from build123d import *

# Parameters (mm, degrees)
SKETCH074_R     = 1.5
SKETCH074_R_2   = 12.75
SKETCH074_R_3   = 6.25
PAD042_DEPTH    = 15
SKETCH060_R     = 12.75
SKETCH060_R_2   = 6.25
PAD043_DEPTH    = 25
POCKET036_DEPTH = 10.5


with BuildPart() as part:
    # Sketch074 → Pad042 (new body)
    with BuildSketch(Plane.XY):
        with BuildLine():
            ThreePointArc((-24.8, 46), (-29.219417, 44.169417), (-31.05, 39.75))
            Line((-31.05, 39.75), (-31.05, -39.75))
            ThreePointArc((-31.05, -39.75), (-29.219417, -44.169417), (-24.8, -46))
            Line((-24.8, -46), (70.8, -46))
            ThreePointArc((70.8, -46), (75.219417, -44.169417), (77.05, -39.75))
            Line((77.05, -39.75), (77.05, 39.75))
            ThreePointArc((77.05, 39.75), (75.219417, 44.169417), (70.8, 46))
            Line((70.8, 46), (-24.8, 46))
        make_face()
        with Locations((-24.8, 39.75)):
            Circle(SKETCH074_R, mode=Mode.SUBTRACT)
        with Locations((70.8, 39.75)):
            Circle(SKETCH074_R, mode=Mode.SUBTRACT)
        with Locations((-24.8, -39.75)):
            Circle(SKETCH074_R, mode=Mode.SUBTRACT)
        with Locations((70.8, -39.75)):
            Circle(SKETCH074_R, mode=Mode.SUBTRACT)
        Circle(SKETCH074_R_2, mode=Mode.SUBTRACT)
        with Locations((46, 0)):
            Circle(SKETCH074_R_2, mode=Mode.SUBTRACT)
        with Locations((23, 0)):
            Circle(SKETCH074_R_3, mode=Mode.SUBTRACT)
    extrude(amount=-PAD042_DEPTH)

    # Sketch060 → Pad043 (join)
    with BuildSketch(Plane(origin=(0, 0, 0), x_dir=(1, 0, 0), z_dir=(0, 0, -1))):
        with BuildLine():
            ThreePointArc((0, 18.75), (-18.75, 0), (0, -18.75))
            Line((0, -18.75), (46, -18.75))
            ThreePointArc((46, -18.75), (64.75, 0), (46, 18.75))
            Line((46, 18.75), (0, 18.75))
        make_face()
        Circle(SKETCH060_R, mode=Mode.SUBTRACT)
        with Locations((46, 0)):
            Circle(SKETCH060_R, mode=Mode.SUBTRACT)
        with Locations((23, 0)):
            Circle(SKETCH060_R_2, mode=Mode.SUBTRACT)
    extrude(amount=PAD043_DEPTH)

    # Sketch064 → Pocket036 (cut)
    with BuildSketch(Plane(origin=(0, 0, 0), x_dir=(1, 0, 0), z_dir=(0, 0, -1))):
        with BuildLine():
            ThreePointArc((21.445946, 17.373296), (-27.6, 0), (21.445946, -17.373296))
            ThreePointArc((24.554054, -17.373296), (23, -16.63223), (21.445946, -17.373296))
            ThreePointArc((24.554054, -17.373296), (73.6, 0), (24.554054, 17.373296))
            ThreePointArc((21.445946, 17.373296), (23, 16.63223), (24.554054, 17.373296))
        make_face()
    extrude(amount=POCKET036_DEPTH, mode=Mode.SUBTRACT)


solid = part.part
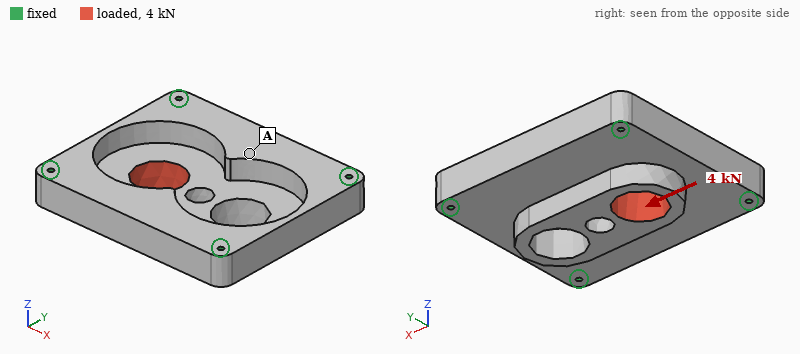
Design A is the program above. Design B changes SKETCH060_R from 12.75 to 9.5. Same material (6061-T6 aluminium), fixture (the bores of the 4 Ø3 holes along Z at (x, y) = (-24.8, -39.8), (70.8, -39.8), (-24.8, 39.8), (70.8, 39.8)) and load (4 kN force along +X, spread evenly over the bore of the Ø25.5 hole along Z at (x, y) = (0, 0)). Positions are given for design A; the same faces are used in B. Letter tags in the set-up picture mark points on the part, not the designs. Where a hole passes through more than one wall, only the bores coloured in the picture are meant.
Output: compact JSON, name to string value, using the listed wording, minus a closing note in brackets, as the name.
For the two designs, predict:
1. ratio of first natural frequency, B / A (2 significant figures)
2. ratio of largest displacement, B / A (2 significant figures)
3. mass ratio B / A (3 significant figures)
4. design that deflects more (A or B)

{"ratio of first natural frequency, B / A": "0.97", "ratio of largest displacement, B / A": "0.78", "mass ratio B / A": "1.06", "design that deflects more": "A"}
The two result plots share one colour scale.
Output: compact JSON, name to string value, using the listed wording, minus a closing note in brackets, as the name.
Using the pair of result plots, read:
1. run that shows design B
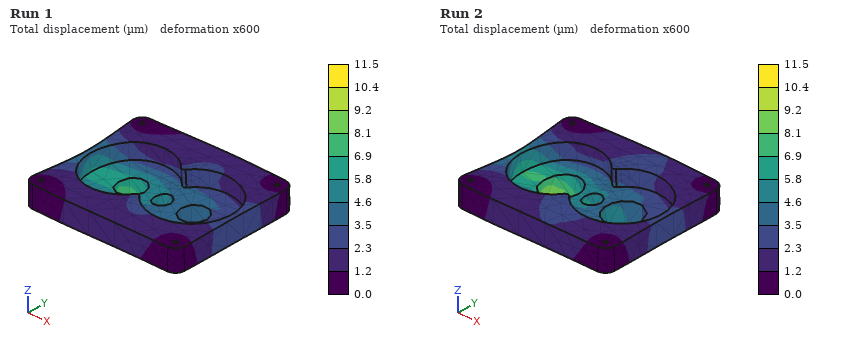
{"run that shows design B": "Run 1"}
